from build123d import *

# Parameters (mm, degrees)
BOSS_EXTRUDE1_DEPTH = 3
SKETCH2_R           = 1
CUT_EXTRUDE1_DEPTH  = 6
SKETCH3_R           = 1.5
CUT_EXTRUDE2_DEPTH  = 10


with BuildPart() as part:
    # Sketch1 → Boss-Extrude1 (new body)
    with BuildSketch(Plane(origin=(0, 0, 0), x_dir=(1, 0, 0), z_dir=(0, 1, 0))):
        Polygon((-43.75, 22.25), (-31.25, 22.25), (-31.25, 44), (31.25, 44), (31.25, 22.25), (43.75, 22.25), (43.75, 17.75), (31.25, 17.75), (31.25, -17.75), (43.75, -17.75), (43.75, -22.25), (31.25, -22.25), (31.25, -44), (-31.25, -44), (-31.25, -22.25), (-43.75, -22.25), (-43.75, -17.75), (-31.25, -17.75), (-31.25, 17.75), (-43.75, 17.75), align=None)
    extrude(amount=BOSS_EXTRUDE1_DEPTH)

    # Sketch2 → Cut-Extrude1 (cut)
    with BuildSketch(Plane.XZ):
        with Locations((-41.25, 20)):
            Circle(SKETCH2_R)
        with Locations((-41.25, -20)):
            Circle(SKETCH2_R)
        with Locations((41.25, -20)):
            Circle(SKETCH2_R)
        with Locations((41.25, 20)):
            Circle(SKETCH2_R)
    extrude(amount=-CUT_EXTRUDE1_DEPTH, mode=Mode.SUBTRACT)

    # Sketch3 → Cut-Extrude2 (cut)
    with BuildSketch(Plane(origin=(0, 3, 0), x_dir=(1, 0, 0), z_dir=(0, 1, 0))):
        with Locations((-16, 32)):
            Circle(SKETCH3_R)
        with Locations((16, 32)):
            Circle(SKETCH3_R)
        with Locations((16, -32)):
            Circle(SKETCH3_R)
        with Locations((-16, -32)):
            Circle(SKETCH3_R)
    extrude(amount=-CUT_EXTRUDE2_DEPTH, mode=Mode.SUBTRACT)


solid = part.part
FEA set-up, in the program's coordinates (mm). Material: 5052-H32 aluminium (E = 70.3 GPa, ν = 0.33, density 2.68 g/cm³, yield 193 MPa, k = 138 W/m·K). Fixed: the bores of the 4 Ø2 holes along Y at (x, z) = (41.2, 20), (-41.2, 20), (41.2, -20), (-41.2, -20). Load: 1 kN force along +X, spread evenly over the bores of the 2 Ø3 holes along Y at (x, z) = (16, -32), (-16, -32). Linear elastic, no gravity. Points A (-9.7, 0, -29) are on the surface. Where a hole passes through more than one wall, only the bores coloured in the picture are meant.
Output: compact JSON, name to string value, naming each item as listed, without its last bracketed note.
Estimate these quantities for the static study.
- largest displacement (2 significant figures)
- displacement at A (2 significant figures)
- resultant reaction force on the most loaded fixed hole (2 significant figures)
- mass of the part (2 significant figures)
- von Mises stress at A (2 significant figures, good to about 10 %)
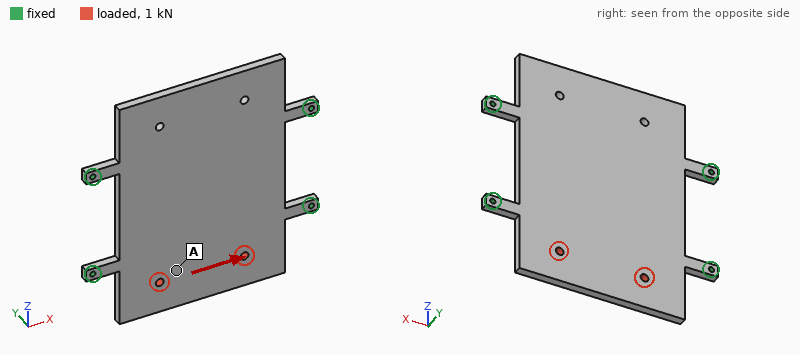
{"largest displacement": "19 µm", "displacement at A": "12 µm", "resultant reaction force on the most loaded fixed hole": "530 N", "mass of the part": "46 g", "von Mises stress at A": "9.6 MPa"}
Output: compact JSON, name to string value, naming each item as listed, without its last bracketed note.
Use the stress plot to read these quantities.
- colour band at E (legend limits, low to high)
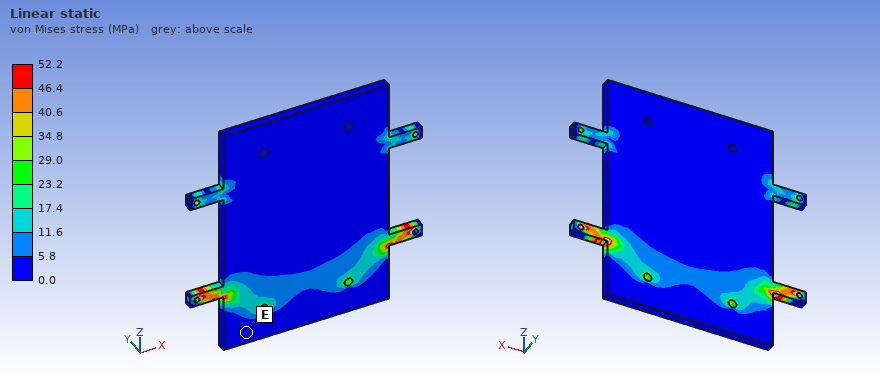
{"colour band at E": "0.0 to 5.8 MPa"}
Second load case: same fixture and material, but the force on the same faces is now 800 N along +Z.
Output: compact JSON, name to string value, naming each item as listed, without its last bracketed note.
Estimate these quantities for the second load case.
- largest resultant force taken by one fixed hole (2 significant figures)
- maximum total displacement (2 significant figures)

{"largest resultant force taken by one fixed hole": "200 N", "maximum total displacement": "28 µm"}
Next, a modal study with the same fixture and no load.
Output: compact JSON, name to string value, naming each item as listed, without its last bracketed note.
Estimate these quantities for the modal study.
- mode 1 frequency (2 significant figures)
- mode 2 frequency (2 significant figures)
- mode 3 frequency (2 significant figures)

{"mode 1 frequency": "1300 Hz", "mode 2 frequency": "1300 Hz", "mode 3 frequency": "2500 Hz"}
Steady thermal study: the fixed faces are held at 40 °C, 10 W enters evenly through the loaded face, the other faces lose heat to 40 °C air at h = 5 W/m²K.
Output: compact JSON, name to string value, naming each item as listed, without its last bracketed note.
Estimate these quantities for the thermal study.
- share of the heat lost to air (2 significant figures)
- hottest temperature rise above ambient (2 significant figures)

{"share of the heat lost to air": "9.8 %", "hottest temperature rise above ambient": "26 K"}
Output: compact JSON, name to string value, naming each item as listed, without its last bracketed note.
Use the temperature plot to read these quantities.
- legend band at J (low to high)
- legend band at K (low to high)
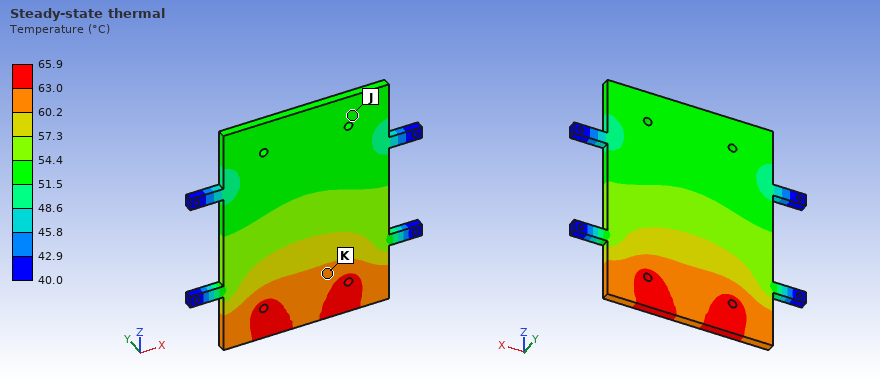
{"legend band at J": "51.5 to 54.4 °C", "legend band at K": "60.2 to 63.0 °C"}
